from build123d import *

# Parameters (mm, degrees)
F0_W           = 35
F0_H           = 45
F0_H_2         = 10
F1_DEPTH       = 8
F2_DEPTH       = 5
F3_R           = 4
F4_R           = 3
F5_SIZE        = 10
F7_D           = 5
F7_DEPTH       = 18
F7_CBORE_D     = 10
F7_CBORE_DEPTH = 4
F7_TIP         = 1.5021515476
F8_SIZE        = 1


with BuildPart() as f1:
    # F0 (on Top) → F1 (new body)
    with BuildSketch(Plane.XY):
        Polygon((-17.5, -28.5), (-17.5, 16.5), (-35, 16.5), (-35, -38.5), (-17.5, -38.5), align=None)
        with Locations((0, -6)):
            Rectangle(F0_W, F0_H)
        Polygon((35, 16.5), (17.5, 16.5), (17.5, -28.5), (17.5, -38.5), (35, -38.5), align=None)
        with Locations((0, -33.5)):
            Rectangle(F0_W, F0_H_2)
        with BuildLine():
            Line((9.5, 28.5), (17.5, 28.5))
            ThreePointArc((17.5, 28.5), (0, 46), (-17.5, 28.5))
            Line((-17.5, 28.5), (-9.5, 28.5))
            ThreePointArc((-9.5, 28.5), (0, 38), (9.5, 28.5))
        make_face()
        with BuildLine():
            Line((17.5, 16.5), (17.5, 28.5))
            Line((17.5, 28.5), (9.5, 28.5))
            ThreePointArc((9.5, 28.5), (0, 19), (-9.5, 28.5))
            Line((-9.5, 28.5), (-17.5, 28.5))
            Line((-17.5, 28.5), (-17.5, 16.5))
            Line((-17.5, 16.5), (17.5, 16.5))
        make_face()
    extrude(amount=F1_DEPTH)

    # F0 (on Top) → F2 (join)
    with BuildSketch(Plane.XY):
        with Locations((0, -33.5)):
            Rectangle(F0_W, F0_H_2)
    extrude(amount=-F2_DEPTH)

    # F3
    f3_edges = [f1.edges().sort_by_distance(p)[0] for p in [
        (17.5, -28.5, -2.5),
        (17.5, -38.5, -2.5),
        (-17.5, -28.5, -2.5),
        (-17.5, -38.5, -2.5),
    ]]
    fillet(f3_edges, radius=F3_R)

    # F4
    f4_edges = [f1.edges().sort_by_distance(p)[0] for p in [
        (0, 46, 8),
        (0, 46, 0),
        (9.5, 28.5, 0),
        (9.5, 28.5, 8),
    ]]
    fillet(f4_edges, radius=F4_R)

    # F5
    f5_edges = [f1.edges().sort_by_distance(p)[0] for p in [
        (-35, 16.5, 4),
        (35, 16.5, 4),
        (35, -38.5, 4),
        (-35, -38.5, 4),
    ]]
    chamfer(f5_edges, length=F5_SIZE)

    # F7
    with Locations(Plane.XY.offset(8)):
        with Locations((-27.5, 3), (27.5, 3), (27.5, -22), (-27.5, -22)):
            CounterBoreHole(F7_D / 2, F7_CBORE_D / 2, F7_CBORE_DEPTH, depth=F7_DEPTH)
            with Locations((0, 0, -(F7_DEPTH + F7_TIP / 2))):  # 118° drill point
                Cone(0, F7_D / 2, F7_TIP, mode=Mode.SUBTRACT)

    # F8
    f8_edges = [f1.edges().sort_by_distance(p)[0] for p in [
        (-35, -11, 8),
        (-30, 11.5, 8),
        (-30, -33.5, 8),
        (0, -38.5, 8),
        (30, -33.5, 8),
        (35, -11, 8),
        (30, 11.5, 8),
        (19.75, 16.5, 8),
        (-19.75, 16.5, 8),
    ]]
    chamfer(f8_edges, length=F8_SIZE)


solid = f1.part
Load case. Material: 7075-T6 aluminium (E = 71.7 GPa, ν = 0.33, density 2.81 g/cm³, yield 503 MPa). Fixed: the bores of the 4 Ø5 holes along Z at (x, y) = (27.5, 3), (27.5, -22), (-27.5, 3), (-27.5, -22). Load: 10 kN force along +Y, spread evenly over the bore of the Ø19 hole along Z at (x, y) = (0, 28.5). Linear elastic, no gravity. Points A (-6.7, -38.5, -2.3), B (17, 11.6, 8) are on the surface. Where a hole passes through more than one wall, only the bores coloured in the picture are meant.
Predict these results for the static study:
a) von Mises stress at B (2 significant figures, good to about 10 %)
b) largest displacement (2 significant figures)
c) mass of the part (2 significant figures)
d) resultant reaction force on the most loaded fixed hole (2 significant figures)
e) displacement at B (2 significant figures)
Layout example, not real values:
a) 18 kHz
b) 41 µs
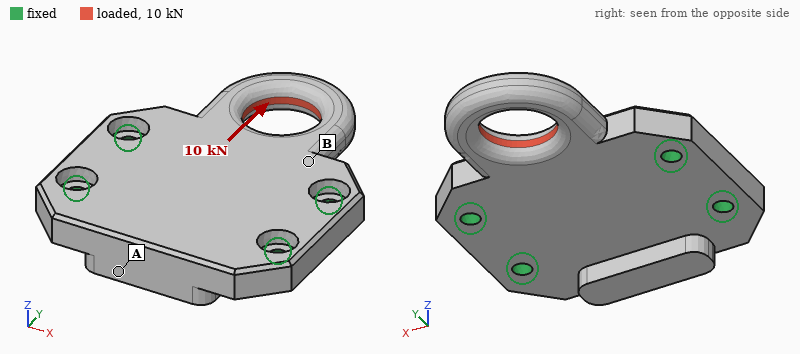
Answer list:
a) 42 MPa
b) 54 µm
c) 94 g
d) 2.9 kN
e) 17 µm
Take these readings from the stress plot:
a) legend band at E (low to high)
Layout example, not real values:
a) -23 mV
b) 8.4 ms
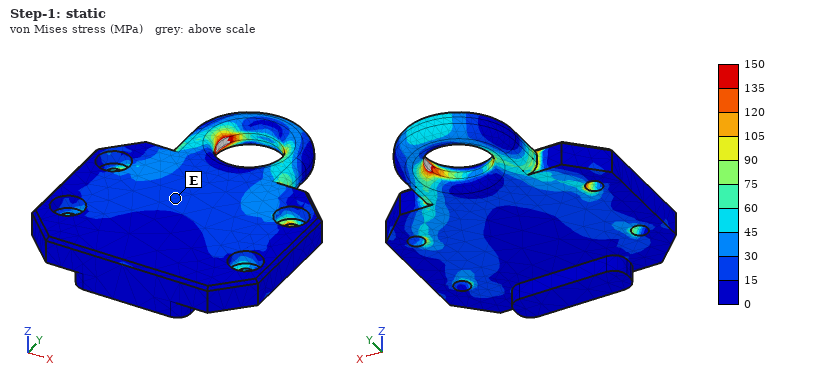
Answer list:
a) 15 to 30 MPa
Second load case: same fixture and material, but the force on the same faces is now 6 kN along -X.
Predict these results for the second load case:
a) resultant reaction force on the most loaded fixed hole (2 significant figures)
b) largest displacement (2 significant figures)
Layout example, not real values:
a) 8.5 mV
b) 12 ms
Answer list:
a) 3.4 kN
b) 0.10 mm
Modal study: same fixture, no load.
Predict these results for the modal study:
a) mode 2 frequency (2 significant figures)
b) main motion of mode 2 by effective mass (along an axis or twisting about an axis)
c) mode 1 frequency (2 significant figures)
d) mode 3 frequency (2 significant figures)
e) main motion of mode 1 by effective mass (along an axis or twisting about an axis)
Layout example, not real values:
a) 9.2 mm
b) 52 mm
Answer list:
a) 7900 Hz
b) along Z
c) 3500 Hz
d) 9900 Hz
e) along Z
